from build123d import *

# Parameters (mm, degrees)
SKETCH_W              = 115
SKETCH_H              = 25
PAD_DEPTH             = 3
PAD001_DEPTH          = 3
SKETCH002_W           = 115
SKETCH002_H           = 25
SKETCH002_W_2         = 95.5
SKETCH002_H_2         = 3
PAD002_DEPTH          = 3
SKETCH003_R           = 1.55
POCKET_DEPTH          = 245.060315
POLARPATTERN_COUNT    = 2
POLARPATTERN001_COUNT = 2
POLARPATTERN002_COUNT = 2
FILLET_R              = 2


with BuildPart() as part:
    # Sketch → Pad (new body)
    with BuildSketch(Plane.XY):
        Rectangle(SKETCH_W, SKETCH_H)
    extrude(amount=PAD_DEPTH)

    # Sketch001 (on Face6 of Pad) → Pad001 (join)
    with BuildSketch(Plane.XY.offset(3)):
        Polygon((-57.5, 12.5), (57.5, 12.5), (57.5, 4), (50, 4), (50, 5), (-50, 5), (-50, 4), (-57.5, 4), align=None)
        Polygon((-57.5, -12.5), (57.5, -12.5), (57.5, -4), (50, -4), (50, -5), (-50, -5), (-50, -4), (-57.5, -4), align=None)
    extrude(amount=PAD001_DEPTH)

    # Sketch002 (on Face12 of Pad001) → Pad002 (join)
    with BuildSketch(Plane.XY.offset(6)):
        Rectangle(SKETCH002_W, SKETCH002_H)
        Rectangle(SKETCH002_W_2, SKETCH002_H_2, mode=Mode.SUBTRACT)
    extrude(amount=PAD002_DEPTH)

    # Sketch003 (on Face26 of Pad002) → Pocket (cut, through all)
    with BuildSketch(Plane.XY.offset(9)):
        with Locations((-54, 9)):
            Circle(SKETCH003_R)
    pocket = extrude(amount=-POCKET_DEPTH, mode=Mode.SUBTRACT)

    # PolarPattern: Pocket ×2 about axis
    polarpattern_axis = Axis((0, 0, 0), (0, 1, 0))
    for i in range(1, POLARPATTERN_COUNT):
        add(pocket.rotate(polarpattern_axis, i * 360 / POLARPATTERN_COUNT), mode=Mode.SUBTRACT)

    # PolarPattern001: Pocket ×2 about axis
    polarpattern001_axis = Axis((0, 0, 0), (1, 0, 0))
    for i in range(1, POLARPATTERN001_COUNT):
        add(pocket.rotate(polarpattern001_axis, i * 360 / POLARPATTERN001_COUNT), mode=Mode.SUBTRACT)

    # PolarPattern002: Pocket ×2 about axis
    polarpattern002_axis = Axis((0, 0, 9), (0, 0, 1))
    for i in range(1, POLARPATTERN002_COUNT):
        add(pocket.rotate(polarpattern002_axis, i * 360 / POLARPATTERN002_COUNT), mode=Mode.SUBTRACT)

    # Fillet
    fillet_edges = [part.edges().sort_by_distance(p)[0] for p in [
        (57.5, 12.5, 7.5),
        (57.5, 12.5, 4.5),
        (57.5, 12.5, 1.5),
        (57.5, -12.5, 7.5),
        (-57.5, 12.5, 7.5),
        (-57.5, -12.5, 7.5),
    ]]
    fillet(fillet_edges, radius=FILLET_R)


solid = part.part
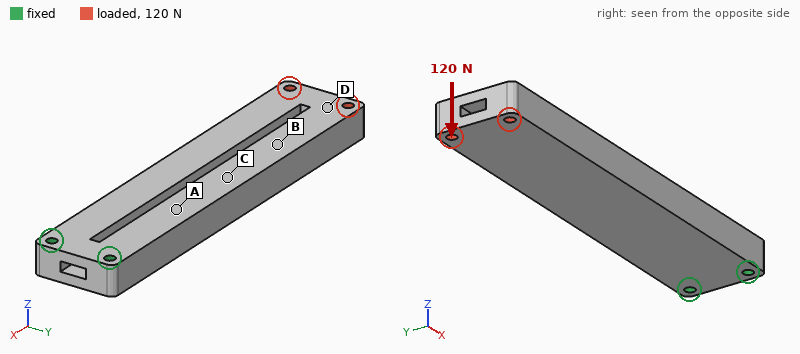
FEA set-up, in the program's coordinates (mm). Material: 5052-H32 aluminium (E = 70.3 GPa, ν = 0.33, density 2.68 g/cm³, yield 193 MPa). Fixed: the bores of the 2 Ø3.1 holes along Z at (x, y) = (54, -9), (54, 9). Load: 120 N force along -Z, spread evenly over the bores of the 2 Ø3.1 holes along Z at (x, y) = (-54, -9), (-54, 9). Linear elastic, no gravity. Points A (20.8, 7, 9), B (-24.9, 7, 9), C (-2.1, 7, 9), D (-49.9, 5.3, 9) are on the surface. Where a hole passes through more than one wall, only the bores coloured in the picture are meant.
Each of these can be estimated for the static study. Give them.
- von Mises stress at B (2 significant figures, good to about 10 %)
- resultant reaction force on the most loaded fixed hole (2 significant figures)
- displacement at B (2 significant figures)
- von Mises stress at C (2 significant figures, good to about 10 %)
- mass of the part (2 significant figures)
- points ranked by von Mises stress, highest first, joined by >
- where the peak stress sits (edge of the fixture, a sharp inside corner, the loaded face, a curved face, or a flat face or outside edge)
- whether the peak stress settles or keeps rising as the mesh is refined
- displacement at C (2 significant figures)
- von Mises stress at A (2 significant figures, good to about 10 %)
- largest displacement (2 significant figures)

12 MPa
69 N
0.33 mm
21 MPa
57 g
A > C > B > D
edge of the fixture
keeps rising
0.18 mm
30 MPa
0.56 mm
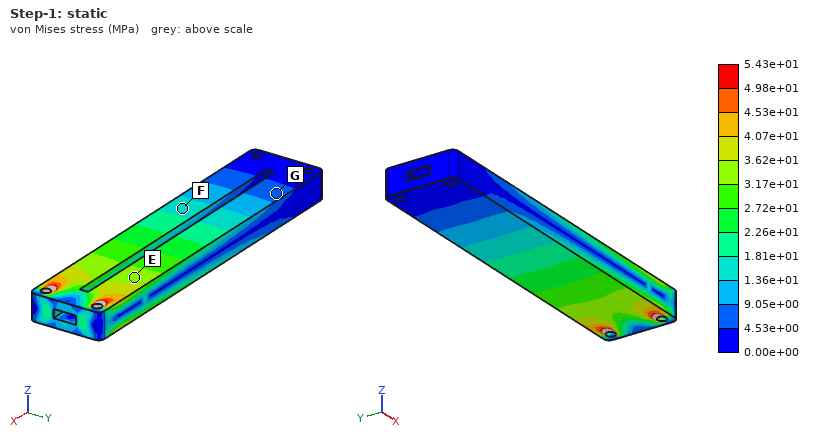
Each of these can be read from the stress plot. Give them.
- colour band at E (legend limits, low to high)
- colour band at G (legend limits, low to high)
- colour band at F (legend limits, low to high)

3.17e+01 to 3.62e+01 MPa
4.53e+00 to 9.05e+00 MPa
1.36e+01 to 1.81e+01 MPa
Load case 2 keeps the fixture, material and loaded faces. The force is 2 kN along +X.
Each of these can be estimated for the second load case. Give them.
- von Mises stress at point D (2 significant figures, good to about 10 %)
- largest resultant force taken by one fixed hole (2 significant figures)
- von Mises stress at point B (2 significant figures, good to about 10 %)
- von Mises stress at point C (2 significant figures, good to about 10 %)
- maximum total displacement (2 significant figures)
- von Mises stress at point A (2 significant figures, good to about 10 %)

9.2 MPa
1.0 kN
12 MPa
12 MPa
25 µm
12 MPa
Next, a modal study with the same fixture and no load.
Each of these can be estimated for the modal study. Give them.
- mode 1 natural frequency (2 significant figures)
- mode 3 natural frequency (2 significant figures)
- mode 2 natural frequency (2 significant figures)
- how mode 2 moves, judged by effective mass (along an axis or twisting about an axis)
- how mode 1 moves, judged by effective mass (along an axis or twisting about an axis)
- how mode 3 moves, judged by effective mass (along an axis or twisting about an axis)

620 Hz
3100 Hz
1600 Hz
along Y
along Z
twisting about X
